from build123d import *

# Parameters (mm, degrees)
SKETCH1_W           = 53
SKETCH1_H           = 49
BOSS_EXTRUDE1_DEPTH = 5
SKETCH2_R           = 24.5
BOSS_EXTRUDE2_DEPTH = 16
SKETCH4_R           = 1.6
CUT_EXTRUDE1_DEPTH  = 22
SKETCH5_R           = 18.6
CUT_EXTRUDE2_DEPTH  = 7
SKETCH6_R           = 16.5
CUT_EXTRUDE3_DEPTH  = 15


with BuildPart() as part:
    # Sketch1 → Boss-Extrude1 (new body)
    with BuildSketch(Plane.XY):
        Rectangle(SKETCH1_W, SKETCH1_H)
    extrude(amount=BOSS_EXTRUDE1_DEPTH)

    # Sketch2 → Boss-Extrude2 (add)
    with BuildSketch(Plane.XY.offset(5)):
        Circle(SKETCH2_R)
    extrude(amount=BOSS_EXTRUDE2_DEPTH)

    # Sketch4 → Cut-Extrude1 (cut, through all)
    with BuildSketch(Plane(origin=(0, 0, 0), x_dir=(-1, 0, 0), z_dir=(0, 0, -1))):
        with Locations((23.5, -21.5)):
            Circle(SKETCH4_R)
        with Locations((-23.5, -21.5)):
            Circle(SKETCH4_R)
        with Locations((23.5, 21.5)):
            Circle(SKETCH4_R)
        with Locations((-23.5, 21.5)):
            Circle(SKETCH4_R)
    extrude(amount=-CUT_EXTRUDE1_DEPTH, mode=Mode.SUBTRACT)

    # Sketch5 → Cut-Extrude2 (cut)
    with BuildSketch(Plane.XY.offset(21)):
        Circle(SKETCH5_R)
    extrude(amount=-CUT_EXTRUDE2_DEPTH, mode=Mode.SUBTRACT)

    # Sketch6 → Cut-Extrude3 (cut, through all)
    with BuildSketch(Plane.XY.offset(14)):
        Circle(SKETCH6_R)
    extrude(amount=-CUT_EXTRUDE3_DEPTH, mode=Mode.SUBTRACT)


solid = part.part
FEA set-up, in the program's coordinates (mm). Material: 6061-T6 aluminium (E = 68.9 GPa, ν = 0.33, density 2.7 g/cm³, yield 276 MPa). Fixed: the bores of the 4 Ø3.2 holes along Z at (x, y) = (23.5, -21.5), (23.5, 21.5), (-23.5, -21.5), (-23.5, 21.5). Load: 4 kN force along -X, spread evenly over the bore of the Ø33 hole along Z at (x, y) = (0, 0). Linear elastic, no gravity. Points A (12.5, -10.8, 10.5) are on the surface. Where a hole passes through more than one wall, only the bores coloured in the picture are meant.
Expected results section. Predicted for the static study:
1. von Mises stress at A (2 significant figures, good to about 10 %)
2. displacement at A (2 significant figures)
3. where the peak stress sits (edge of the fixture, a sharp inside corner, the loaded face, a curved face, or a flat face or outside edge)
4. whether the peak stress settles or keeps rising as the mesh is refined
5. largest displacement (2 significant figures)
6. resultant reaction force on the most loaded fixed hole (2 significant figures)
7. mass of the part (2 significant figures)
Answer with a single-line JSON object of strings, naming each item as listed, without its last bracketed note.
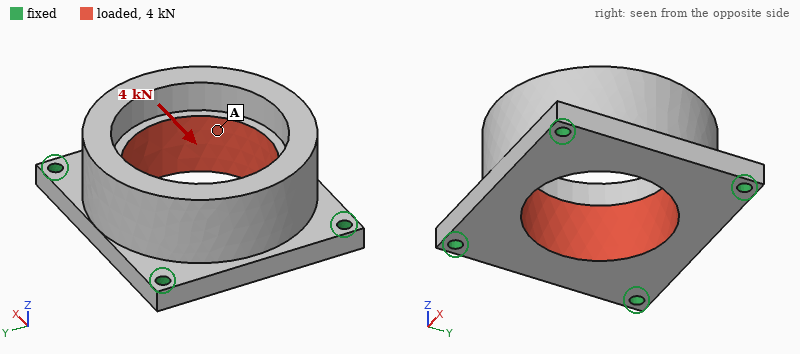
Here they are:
{"von Mises stress at A": "8.0 MPa", "displacement at A": "6.9 µm", "where the peak stress sits": "edge of the fixture", "whether the peak stress settles or keeps rising as the mesh is refined": "keeps rising", "largest displacement": "9.2 µm", "resultant reaction force on the most loaded fixed hole": "1.1 kN", "mass of the part": "63 g"}
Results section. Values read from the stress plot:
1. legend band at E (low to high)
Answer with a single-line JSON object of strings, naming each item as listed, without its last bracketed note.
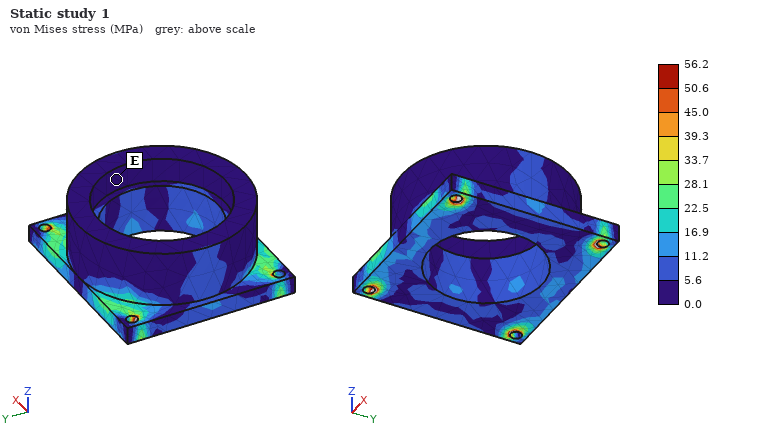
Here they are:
{"legend band at E": "0.0 to 5.6 MPa"}
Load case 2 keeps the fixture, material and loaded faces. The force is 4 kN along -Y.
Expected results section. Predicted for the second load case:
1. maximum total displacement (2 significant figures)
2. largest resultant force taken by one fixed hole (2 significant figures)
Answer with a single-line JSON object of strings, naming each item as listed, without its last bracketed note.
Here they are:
{"maximum total displacement": "10 µm", "largest resultant force taken by one fixed hole": "1.1 kN"}
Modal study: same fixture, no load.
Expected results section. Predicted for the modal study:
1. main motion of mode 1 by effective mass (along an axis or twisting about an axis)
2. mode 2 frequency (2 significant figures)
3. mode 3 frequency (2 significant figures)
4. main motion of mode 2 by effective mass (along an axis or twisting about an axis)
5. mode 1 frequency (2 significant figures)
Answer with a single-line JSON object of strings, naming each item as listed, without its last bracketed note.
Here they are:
{"main motion of mode 1 by effective mass": "along Z", "mode 2 frequency": "11 kHz", "mode 3 frequency": "12 kHz", "main motion of mode 2 by effective mass": "along Y", "mode 1 frequency": "10 kHz"}
